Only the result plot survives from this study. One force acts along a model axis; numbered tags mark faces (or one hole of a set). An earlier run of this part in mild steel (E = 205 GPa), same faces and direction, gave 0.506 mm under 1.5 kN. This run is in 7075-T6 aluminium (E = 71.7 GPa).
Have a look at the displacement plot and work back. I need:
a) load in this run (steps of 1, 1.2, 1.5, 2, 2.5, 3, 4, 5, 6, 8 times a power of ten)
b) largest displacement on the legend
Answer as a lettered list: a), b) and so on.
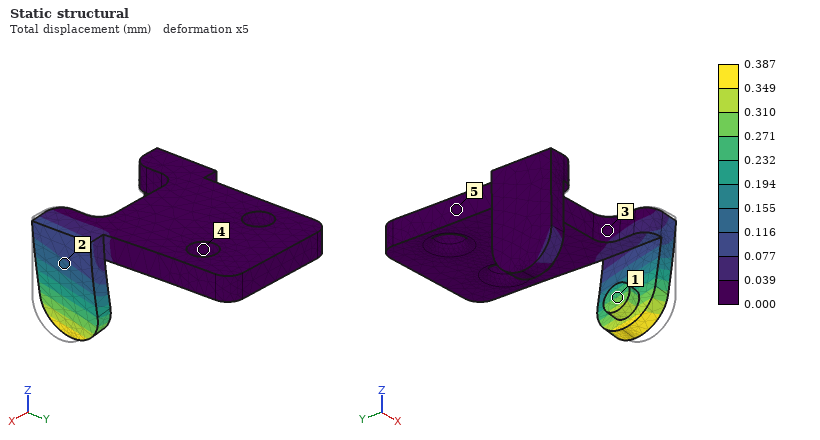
a) 400 N
b) 0.387 mm
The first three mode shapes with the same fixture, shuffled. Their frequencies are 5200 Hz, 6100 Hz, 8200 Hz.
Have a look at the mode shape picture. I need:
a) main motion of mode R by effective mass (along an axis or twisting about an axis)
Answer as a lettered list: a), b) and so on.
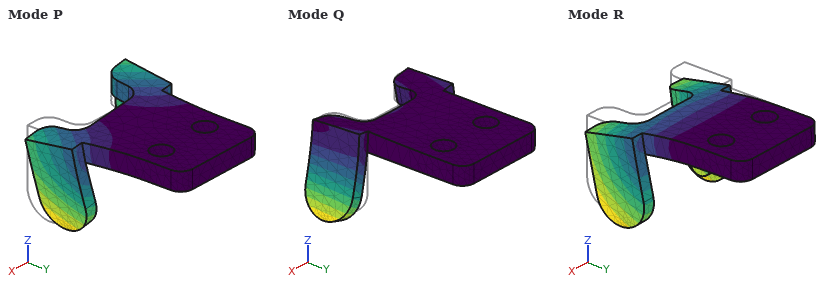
a) along Z
